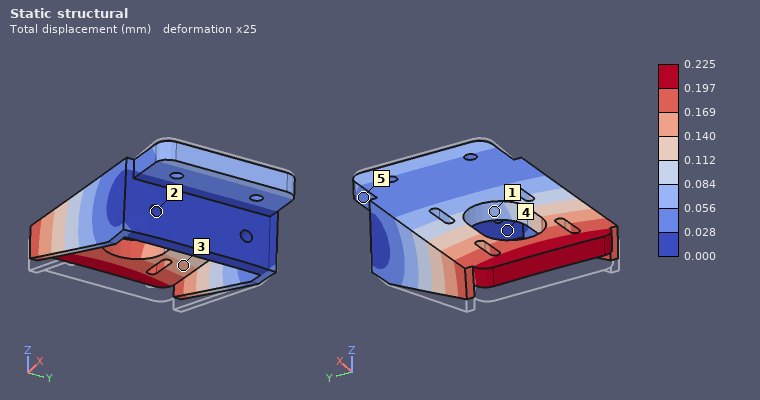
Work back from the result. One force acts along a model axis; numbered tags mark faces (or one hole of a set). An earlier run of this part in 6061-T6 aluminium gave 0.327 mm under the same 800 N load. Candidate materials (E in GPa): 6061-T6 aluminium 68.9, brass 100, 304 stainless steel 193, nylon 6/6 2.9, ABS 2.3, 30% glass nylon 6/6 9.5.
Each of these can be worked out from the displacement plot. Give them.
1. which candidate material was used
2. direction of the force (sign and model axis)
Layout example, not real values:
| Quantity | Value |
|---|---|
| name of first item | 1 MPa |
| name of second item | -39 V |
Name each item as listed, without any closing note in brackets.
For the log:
| Quantity | Value |
|---|---|
| which candidate material was used | brass |
| direction of the force | +Z |
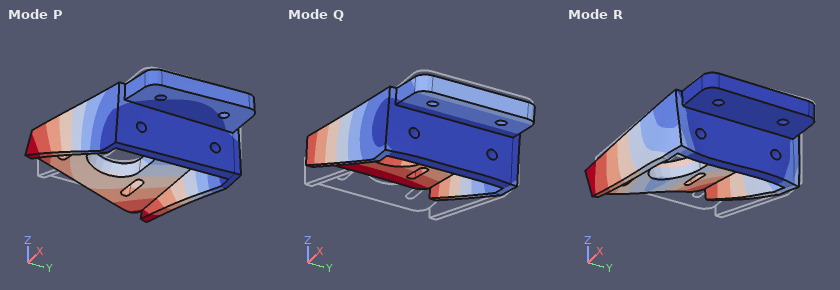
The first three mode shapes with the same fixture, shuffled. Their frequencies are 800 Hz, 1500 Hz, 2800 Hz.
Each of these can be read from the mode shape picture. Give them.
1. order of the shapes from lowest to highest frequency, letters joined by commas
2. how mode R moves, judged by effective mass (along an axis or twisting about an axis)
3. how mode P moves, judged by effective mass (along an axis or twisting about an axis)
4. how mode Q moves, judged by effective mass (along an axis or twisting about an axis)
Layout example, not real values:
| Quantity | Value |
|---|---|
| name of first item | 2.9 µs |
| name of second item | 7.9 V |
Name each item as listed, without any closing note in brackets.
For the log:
| Quantity | Value |
|---|---|
| order of the shapes from lowest to highest frequency, letters joined by commas | Q, P, R |
| how mode R moves, judged by effective mass | along Y |
| how mode P moves, judged by effective mass | along Y |
| how mode Q moves, judged by effective mass | along Z |
